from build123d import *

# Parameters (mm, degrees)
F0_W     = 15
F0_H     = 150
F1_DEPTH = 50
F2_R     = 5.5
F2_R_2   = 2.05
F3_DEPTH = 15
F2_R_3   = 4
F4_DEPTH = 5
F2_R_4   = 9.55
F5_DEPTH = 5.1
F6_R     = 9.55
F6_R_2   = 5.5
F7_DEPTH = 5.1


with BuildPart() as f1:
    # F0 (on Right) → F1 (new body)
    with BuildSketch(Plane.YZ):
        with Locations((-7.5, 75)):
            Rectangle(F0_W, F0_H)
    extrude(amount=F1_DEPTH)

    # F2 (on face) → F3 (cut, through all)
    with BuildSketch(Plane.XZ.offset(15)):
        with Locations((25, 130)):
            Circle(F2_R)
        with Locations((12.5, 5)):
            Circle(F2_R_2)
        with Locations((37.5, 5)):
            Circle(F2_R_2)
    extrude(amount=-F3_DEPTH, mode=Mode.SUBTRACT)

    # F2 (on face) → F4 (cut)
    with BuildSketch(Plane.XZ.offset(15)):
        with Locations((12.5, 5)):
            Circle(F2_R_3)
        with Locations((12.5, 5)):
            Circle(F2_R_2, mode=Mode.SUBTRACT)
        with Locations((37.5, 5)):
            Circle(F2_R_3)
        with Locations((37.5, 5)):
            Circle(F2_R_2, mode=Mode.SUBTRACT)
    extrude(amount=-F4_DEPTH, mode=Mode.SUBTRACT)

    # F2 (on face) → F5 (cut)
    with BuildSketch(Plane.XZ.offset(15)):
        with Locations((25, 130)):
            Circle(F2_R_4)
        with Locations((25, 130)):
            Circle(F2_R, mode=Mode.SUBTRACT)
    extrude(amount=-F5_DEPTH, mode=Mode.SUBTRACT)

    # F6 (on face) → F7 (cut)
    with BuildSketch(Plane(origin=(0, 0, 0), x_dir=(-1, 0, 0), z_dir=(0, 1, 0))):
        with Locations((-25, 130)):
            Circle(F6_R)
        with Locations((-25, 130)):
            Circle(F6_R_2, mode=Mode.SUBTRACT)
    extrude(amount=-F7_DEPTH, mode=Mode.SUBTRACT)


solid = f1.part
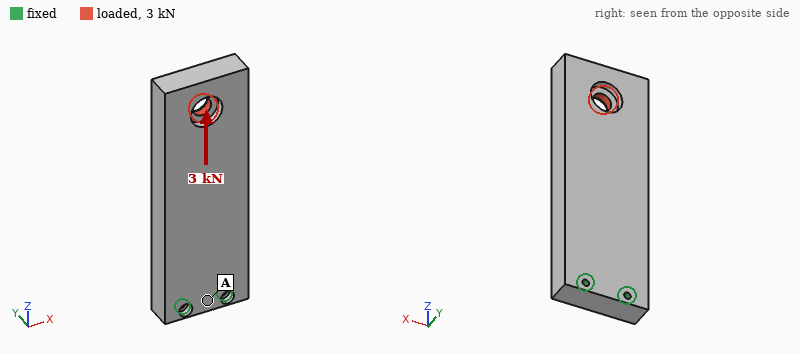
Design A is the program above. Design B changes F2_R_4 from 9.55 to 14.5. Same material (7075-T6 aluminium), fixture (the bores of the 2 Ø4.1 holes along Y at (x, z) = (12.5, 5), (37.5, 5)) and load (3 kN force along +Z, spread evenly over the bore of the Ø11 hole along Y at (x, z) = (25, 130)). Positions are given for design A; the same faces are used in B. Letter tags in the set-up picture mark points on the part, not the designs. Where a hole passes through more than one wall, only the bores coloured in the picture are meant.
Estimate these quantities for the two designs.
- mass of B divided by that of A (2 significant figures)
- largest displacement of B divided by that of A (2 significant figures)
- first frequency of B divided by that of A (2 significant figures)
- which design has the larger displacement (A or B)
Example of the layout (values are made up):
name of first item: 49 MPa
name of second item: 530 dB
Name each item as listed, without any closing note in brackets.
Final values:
mass of B divided by that of A: 0.98
largest displacement of B divided by that of A: 1.1
first frequency of B divided by that of A: 1.0
which design has the larger displacement: B
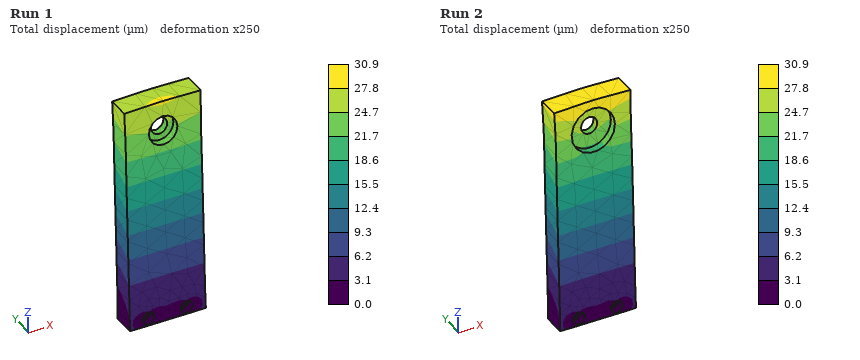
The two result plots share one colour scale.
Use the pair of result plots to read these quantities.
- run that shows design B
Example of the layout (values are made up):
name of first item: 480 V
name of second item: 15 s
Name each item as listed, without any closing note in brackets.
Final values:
run that shows design B: Run 2
